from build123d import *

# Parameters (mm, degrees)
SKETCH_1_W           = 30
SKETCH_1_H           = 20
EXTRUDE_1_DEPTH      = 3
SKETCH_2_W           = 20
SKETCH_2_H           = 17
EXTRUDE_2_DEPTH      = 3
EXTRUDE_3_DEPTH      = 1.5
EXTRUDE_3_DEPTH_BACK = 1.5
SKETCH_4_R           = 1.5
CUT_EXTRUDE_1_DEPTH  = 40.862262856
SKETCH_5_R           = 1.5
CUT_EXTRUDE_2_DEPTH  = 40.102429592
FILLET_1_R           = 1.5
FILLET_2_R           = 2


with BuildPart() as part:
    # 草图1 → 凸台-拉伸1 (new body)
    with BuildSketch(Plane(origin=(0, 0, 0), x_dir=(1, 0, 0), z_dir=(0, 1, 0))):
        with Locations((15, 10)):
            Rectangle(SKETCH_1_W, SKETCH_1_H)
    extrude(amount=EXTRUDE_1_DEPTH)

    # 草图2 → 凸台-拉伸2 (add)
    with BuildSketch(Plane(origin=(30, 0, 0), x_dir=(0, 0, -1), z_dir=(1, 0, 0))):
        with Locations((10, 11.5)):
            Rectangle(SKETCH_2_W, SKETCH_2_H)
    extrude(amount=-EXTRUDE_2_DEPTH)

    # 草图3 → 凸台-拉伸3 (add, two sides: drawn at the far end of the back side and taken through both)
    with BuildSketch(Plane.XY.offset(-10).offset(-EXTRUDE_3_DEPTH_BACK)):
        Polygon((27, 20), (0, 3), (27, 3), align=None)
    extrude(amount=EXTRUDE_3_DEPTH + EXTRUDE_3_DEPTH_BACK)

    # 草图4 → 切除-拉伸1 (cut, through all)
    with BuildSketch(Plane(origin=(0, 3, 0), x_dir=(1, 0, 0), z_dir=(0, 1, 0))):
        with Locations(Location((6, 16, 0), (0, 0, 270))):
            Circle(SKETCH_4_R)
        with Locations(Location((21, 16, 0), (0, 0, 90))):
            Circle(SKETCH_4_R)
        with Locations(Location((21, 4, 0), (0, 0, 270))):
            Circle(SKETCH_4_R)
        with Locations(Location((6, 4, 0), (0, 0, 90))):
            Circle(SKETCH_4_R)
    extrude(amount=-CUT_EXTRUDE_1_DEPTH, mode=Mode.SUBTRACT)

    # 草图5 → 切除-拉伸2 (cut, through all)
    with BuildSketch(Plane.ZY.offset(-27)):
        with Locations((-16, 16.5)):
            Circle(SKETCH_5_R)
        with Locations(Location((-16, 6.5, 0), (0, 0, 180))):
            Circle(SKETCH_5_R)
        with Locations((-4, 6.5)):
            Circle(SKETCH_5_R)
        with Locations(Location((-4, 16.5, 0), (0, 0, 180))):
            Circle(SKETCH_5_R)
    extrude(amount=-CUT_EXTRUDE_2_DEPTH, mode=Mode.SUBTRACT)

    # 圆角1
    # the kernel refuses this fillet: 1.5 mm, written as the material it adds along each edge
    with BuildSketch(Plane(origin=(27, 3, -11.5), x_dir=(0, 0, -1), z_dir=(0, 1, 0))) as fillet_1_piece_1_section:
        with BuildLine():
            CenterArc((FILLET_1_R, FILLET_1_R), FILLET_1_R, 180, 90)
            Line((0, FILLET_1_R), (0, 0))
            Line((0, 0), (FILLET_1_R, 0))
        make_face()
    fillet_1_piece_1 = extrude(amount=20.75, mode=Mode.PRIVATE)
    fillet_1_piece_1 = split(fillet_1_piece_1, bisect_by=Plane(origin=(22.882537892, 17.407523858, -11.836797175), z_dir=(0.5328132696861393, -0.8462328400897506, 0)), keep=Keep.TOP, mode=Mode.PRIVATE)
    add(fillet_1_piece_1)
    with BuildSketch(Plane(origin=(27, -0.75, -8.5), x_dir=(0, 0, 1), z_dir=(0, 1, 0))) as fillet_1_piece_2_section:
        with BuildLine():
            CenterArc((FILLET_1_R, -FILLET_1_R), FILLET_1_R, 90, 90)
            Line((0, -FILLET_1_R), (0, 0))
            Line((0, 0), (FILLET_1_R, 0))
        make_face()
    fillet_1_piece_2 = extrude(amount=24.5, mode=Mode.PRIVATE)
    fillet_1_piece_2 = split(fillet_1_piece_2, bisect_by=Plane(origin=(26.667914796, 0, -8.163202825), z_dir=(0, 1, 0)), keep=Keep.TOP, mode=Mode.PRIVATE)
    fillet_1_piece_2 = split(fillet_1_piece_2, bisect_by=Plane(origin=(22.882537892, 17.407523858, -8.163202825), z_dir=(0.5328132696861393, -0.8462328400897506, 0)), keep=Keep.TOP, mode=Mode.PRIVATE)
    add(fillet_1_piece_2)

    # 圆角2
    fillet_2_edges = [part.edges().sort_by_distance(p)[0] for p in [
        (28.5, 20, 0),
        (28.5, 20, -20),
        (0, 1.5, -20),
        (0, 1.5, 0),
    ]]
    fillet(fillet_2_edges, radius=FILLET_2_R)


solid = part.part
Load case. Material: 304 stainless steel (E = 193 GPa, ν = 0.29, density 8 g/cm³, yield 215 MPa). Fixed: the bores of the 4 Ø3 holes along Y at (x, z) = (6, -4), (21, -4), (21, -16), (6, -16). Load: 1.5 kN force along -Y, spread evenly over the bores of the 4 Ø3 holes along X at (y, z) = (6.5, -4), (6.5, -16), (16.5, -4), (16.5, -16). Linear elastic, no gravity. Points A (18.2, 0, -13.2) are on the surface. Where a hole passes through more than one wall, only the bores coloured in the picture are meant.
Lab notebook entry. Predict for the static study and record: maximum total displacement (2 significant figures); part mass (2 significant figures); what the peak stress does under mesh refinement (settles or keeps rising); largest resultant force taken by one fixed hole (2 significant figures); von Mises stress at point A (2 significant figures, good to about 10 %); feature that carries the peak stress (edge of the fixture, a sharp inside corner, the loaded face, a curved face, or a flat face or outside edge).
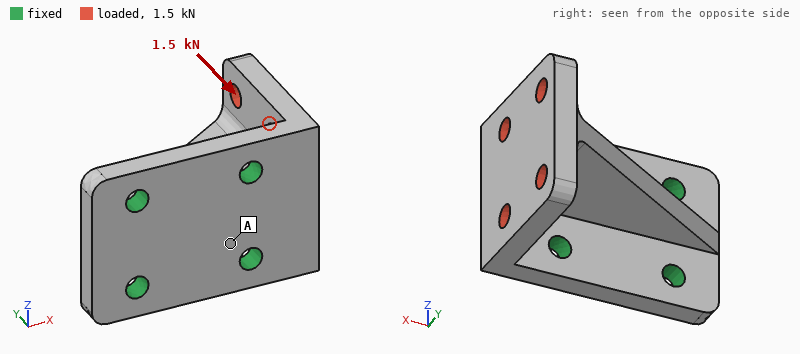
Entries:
16 µm
27 g
keeps rising
980 N
27 MPa
edge of the fixture
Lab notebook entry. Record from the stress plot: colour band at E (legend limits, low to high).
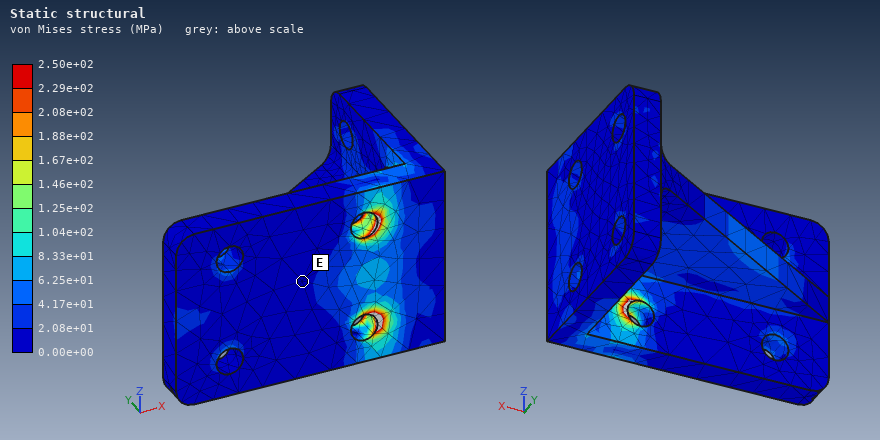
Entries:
0.00e+00 to 2.08e+01 MPa
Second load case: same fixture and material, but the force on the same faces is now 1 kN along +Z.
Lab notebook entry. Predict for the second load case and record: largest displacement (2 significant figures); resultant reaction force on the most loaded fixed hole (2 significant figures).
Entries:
28 µm
1.0 kN
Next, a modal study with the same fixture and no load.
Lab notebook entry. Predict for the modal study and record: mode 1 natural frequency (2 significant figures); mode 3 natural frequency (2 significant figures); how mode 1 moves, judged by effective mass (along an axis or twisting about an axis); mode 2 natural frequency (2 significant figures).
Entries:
11 kHz
18 kHz
along Z
14 kHz
